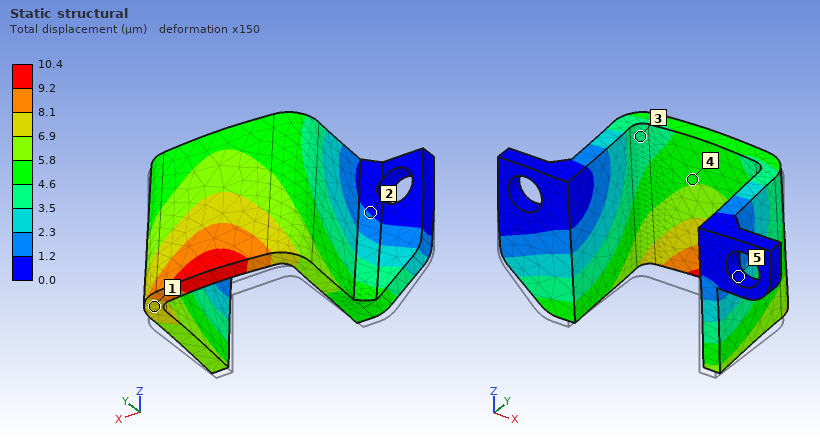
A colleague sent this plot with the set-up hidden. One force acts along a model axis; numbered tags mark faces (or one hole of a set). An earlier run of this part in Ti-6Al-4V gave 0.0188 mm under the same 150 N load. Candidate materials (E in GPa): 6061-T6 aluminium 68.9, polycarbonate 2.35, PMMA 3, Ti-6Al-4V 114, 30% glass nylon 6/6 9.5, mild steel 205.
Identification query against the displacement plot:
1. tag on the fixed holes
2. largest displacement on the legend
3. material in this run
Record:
5
10.4 µm
mild steel
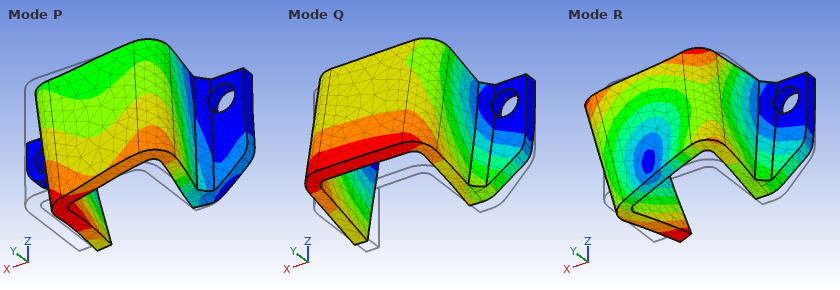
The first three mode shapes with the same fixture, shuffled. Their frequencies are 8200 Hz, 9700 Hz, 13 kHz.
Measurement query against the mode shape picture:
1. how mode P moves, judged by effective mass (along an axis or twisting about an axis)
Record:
along X
